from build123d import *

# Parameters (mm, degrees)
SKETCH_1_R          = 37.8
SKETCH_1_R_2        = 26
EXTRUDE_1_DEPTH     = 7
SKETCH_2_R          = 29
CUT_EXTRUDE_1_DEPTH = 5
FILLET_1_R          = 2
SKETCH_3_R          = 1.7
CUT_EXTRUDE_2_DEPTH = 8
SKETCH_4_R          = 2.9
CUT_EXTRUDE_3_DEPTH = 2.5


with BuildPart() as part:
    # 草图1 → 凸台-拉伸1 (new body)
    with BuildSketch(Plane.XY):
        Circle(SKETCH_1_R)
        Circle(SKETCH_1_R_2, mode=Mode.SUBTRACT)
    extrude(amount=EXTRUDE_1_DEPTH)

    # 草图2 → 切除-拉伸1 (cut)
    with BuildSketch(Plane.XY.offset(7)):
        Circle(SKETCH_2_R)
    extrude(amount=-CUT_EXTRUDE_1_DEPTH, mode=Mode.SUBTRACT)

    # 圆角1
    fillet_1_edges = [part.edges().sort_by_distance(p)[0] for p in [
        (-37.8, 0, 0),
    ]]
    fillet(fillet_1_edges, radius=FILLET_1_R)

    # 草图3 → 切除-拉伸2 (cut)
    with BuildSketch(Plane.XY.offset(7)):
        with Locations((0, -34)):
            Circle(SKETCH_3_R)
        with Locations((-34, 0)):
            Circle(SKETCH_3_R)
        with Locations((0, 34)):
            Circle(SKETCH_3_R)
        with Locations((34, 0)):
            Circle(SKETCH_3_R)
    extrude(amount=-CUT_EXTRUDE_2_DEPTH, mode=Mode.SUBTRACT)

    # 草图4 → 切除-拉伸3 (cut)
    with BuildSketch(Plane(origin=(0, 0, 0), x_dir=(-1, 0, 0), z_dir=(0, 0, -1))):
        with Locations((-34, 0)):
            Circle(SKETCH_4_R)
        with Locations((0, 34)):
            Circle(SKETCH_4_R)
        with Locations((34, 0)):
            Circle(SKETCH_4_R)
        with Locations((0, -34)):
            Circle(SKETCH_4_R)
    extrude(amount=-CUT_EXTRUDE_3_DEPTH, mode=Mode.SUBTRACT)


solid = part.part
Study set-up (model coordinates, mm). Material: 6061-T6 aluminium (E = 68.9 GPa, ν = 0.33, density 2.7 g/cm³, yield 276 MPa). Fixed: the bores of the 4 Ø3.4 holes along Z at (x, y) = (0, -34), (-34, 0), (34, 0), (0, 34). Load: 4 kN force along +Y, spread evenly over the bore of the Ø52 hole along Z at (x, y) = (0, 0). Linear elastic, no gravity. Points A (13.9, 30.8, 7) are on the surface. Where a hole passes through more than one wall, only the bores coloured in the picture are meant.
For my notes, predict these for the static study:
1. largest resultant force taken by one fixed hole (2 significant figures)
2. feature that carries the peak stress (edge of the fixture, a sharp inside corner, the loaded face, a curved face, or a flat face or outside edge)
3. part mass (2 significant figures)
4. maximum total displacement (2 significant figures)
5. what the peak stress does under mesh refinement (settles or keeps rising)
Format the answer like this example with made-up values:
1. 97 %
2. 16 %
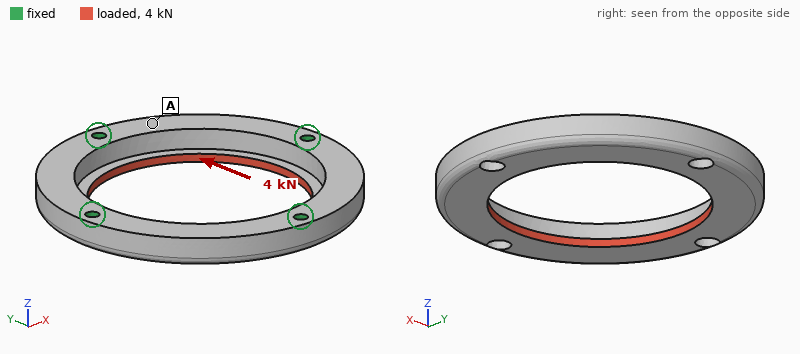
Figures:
1. 1.3 kN
2. edge of the fixture
3. 36 g
4. 14 µm
5. keeps rising
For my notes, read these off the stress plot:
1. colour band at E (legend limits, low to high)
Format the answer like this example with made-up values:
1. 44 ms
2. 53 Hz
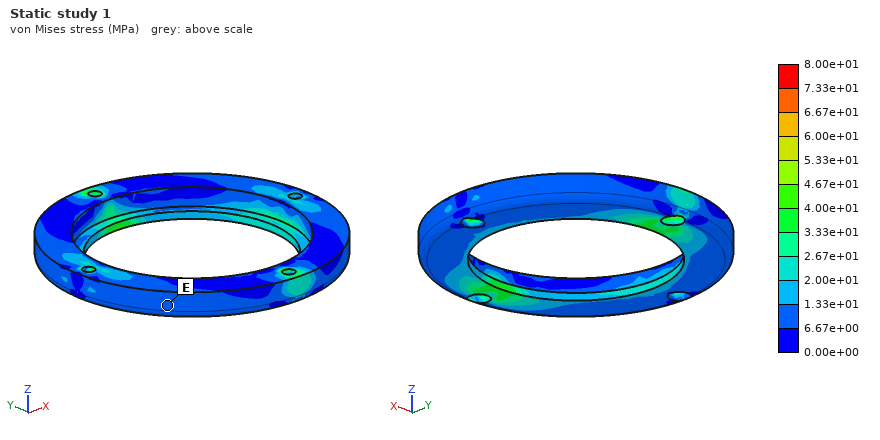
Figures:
1. 6.67e+00 to 1.33e+01 MPa
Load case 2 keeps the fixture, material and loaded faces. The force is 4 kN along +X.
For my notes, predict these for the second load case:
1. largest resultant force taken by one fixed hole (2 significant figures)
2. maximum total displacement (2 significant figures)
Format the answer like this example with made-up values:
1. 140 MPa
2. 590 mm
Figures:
1. 1.3 kN
2. 14 µm
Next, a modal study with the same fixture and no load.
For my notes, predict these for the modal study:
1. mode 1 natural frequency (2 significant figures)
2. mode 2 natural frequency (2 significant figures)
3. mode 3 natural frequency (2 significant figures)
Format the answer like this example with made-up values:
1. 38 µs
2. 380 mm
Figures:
1. 8600 Hz
2. 9700 Hz
3. 9700 Hz
